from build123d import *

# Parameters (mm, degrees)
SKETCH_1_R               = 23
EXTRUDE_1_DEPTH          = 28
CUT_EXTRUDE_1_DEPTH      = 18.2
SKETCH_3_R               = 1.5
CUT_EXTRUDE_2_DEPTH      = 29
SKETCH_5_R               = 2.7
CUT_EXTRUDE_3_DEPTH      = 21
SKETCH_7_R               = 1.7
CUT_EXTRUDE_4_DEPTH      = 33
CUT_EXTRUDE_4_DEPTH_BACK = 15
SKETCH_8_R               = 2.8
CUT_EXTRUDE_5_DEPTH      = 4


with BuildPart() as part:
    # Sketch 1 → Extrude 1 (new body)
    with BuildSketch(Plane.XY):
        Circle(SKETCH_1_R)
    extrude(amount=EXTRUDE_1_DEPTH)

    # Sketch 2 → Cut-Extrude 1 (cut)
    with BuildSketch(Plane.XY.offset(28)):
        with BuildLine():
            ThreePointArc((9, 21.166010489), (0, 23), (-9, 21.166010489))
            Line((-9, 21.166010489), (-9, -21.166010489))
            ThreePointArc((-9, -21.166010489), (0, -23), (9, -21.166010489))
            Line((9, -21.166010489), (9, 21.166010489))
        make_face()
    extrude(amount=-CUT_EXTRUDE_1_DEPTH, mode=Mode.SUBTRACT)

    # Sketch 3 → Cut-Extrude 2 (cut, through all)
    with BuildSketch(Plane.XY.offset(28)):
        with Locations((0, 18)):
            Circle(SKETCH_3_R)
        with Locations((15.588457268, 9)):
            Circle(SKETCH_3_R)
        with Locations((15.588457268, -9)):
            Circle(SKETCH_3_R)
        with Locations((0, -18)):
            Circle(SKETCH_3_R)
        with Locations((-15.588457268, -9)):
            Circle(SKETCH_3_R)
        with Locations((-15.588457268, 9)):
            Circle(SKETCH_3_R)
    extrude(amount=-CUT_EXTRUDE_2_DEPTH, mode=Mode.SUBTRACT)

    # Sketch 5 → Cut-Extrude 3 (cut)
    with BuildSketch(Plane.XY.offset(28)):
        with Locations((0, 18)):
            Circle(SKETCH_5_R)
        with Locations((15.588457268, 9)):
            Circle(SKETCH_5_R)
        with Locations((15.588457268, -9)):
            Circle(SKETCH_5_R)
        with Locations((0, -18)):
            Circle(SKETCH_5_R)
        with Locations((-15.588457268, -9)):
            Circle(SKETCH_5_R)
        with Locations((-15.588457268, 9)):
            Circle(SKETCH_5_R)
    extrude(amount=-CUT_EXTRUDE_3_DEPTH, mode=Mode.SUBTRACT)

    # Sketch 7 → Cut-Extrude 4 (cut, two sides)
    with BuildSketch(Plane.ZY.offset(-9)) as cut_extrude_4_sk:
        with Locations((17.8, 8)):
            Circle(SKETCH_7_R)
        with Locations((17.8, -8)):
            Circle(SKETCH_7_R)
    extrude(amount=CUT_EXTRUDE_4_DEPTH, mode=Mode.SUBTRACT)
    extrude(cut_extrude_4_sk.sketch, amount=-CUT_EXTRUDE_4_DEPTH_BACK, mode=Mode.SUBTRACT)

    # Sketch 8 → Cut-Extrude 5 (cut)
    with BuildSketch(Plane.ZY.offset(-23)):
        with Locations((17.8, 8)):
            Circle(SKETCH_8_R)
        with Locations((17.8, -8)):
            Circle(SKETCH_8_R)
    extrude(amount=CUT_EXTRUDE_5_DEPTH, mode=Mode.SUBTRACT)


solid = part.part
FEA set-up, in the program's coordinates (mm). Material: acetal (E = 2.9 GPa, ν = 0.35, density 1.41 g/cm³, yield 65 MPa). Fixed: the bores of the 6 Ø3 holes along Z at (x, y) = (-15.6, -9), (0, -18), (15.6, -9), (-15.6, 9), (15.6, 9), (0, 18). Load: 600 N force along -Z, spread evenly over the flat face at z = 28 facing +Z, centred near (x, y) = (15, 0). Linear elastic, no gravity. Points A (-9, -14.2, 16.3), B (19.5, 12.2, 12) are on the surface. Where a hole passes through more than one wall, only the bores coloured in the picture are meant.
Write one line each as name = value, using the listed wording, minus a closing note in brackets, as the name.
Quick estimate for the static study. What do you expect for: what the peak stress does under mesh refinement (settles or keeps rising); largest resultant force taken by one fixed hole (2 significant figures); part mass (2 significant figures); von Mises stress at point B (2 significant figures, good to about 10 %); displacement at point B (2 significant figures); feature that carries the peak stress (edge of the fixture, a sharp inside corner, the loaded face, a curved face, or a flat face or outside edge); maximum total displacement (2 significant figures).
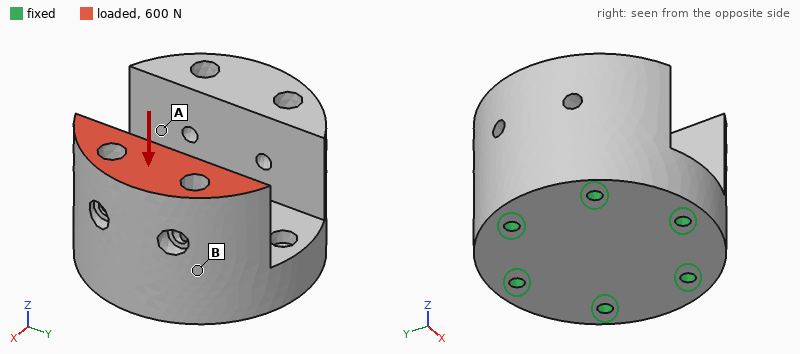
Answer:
what the peak stress does under mesh refinement = keeps rising
largest resultant force taken by one fixed hole = 260 N
part mass = 41 g
von Mises stress at point B = 2.2 MPa
displacement at point B = 13 µm
feature that carries the peak stress = edge of the fixture
maximum total displacement = 29 µm
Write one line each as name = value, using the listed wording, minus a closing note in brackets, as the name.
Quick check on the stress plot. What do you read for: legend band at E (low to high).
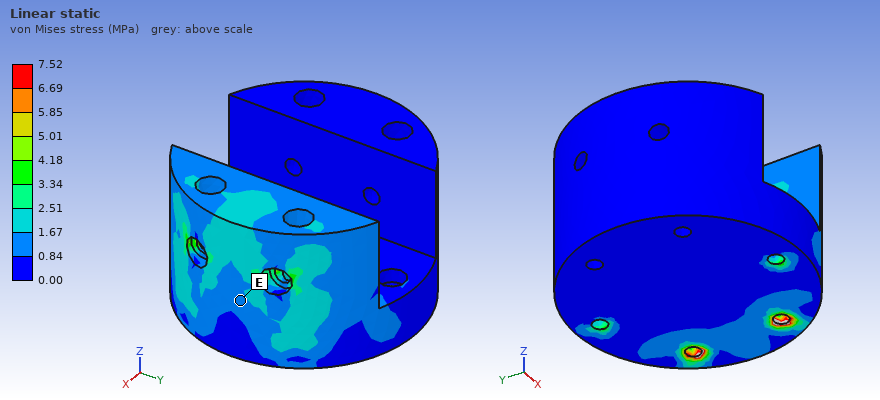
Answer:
legend band at E = 0.84 to 1.67 MPa
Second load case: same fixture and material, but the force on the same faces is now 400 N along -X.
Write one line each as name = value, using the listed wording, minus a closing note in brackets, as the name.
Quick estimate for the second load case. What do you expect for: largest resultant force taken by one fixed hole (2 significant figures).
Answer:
largest resultant force taken by one fixed hole = 220 N
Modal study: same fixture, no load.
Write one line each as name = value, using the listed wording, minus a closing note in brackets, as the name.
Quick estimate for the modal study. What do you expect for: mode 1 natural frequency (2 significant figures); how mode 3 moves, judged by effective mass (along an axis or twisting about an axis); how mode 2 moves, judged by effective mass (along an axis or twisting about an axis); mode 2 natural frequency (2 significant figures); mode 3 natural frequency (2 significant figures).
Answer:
mode 1 natural frequency = 3600 Hz
how mode 3 moves, judged by effective mass = along Y
how mode 2 moves, judged by effective mass = along X
mode 2 natural frequency = 3800 Hz
mode 3 natural frequency = 5400 Hz
